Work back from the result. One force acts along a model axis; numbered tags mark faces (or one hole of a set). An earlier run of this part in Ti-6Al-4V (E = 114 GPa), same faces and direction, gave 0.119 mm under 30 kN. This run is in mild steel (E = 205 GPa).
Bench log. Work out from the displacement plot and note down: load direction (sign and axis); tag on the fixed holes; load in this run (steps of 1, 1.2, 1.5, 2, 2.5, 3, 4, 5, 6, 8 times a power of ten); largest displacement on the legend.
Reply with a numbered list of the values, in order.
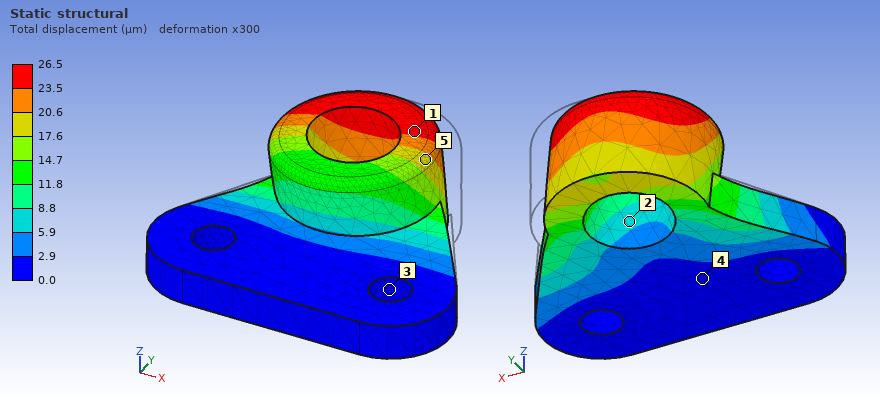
1. -X
2. 3
3. 12 kN
4. 26.5 µm
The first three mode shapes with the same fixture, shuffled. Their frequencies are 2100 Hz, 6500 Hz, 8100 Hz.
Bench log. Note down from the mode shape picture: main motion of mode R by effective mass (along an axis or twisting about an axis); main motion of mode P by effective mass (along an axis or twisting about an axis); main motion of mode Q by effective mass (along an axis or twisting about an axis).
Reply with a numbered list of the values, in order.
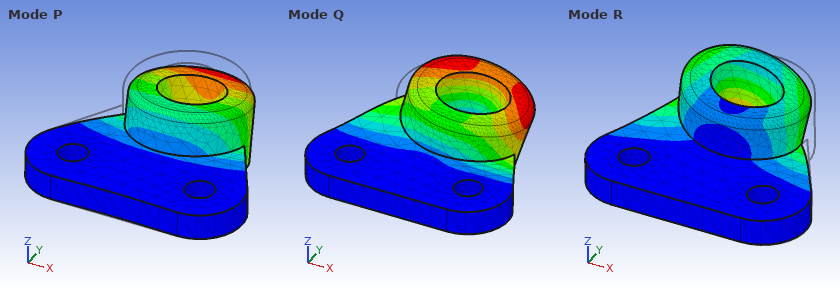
1. along X
2. along Z
3. along X
